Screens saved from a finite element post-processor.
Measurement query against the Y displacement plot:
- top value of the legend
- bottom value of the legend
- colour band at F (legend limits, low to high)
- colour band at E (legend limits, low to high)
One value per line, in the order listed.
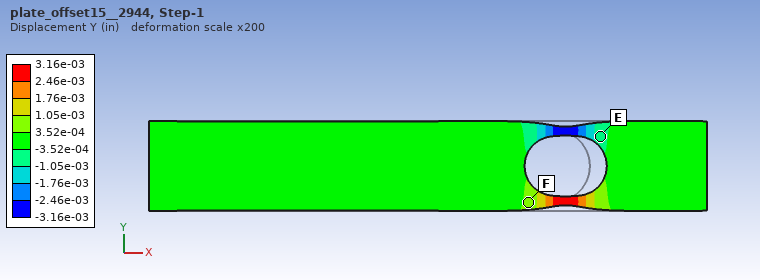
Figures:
3.16e-03 in
-3.16e-03 in
3.52e-04 to 1.05e-03 in
-1.05e-03 to -3.52e-04 in
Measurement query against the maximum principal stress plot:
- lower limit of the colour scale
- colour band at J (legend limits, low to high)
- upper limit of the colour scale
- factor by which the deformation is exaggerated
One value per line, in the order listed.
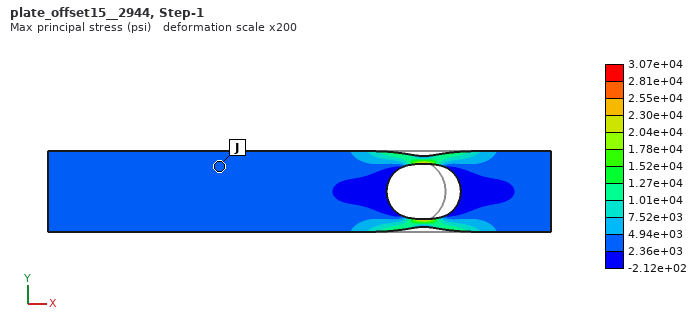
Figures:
-2.12e+02 psi
2.36e+03 to 4.94e+03 psi
3.07e+04 psi
200
